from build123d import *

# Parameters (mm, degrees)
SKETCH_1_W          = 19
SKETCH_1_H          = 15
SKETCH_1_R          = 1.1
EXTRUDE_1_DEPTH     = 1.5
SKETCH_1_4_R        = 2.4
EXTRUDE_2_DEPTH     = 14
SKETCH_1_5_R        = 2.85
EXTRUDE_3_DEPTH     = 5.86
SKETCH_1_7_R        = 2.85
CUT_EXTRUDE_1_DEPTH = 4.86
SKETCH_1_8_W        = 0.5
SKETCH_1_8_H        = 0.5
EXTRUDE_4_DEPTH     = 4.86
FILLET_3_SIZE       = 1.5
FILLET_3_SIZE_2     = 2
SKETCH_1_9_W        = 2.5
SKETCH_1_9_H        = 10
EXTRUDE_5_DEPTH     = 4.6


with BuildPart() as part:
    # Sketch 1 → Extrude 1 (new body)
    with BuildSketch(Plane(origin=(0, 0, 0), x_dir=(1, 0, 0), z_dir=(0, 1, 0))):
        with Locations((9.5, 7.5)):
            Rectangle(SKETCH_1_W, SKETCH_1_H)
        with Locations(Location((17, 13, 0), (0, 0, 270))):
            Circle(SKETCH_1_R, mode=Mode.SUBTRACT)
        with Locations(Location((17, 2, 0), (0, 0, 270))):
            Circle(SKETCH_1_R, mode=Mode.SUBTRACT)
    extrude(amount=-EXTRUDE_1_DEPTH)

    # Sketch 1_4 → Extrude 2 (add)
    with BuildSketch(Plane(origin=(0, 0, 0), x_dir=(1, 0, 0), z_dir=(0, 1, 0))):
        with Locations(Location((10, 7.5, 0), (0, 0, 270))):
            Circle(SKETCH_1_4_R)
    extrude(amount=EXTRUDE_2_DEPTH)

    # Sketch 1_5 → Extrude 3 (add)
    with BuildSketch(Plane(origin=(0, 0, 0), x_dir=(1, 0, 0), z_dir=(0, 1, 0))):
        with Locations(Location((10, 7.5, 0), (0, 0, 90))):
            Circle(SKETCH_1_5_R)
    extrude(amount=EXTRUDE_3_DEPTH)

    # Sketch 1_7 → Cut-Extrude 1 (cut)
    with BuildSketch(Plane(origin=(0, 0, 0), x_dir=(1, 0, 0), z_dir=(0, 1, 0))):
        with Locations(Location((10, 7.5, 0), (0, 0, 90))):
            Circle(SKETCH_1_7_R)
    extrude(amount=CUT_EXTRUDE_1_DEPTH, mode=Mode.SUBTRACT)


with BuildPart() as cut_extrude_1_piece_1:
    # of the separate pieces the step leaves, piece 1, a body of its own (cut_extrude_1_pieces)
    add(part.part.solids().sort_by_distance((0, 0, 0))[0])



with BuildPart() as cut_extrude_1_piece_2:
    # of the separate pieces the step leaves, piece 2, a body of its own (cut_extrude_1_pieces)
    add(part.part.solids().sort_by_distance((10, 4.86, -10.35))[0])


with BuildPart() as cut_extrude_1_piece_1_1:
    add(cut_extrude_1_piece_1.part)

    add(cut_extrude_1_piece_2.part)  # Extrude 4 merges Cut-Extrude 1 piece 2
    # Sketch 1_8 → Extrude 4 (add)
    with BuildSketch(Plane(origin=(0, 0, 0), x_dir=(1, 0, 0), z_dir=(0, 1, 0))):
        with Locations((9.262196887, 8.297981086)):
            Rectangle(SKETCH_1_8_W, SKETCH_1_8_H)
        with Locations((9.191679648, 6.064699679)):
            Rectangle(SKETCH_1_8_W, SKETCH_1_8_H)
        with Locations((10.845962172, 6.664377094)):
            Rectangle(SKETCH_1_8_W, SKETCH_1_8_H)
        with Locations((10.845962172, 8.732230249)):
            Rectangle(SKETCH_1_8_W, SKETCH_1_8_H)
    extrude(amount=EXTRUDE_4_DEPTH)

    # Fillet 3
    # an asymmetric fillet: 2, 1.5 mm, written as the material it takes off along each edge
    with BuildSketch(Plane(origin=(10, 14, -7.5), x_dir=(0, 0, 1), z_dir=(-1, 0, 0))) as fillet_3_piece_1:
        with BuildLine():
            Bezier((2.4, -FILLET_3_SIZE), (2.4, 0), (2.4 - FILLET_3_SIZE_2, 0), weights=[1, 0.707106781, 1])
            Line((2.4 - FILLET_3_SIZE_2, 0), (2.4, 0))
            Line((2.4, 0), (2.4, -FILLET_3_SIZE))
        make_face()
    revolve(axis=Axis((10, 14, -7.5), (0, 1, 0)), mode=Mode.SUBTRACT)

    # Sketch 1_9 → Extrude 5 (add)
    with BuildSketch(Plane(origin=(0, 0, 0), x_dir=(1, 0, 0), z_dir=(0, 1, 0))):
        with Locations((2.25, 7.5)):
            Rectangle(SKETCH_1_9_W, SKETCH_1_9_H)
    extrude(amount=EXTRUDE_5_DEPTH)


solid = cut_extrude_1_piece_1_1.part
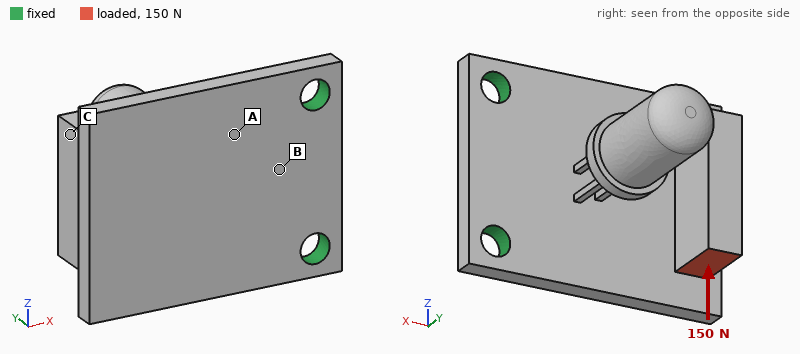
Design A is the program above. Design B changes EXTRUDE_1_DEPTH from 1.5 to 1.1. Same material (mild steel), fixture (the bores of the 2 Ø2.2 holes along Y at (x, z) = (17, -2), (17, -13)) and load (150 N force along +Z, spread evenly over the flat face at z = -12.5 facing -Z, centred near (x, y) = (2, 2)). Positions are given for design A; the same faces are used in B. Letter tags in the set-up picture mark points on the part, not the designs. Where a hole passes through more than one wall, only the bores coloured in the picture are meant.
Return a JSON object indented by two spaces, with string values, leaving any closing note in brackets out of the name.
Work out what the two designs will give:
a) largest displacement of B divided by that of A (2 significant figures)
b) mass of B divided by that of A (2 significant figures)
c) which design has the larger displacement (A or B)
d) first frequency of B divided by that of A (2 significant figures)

{
  "largest displacement of B divided by that of A": "2.1",
  "mass of B divided by that of A": "0.84",
  "which design has the larger displacement": "B",
  "first frequency of B divided by that of A": "0.84"
}
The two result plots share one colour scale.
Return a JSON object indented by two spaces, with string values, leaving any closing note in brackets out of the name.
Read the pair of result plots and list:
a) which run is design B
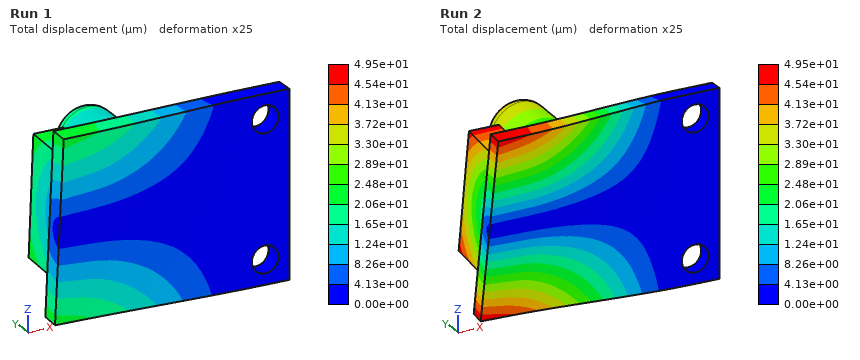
{
  "which run is design B": "Run 2"
}
